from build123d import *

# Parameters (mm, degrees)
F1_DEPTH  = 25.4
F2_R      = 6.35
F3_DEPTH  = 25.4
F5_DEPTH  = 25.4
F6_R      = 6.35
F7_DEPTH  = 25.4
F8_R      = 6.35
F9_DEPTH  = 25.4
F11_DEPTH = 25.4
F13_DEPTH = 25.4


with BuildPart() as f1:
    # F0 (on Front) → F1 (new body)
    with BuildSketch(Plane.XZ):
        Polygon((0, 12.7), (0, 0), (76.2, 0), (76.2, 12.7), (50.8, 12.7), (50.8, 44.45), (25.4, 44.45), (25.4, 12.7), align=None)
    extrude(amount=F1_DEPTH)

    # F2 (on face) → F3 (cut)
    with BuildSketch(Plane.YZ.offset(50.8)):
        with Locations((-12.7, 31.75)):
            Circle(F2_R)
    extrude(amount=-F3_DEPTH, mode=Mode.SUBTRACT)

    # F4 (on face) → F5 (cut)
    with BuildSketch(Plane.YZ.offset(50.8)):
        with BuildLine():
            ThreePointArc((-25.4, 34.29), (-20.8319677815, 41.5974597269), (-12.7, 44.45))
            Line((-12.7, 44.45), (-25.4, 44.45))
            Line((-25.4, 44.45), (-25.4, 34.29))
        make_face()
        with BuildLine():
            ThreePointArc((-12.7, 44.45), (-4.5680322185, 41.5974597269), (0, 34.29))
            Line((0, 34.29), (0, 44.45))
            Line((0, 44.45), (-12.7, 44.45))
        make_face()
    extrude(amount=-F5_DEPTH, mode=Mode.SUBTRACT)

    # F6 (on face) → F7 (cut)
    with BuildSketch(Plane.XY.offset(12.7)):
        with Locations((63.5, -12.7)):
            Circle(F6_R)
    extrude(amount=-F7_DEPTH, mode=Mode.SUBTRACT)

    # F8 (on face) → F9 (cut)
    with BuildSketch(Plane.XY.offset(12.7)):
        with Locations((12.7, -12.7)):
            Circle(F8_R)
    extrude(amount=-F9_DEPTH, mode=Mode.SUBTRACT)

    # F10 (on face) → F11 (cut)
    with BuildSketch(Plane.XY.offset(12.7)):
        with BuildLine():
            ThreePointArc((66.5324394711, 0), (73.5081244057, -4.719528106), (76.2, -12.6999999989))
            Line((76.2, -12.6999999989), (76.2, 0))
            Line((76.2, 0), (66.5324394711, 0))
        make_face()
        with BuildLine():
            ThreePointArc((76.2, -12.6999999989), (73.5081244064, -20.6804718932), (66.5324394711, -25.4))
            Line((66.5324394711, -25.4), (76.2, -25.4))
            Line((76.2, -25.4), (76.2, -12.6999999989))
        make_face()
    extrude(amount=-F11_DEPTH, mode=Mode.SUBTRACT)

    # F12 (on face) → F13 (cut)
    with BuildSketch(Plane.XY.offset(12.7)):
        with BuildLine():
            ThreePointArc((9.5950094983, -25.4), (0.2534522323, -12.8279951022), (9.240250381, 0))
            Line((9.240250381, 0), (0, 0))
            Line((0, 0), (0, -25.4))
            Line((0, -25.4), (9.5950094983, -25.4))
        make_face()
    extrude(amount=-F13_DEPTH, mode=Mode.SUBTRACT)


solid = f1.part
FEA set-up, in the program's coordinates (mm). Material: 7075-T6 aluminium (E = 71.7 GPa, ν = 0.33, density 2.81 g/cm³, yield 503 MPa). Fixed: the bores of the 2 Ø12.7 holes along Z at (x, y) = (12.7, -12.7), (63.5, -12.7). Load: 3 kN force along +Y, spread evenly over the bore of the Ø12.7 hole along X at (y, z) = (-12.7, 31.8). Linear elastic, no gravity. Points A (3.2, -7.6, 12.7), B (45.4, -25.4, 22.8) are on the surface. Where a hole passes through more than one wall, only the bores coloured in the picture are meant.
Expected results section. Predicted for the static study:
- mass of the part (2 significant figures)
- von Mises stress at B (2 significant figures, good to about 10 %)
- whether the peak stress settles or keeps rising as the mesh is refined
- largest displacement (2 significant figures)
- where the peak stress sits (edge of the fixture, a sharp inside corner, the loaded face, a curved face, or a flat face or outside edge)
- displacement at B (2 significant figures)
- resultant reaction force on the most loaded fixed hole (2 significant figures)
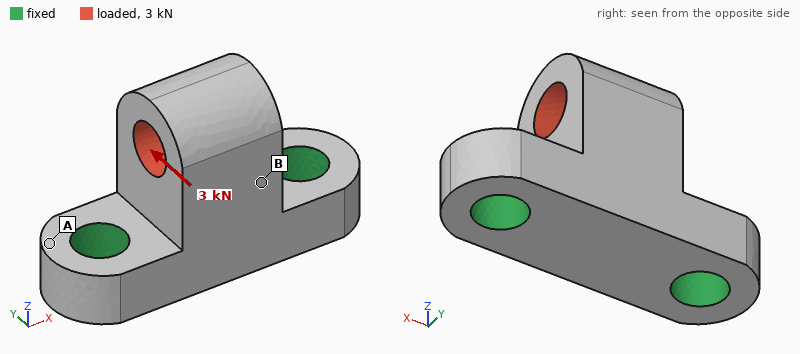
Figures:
99 g
18 MPa
keeps rising
64 µm
edge of the fixture
32 µm
1.5 kN
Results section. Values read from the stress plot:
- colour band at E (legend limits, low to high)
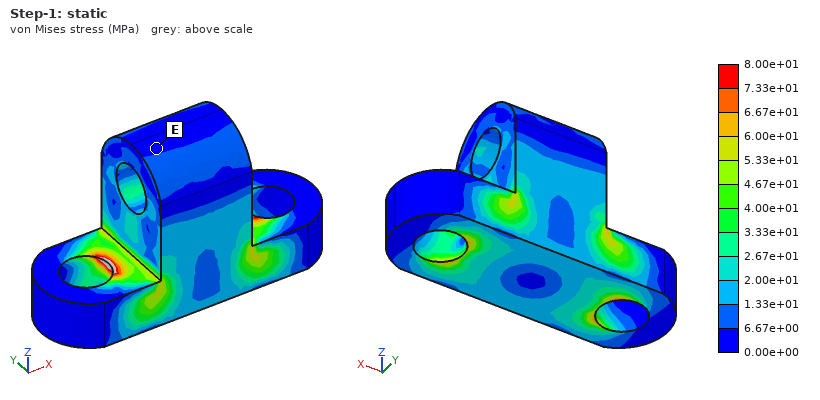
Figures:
0.00e+00 to 6.67e+00 MPa
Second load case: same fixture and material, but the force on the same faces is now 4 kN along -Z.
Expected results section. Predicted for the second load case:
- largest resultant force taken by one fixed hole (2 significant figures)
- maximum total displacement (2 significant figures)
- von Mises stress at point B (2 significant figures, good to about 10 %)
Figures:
2.1 kN
8.8 µm
7.8 MPa
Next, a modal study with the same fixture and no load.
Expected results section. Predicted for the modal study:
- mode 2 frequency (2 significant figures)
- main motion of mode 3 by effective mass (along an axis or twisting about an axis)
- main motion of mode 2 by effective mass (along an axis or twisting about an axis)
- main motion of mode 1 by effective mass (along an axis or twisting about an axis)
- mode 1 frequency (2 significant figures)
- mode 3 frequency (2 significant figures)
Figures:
12 kHz
along Z
along X
along Y
6900 Hz
17 kHz
